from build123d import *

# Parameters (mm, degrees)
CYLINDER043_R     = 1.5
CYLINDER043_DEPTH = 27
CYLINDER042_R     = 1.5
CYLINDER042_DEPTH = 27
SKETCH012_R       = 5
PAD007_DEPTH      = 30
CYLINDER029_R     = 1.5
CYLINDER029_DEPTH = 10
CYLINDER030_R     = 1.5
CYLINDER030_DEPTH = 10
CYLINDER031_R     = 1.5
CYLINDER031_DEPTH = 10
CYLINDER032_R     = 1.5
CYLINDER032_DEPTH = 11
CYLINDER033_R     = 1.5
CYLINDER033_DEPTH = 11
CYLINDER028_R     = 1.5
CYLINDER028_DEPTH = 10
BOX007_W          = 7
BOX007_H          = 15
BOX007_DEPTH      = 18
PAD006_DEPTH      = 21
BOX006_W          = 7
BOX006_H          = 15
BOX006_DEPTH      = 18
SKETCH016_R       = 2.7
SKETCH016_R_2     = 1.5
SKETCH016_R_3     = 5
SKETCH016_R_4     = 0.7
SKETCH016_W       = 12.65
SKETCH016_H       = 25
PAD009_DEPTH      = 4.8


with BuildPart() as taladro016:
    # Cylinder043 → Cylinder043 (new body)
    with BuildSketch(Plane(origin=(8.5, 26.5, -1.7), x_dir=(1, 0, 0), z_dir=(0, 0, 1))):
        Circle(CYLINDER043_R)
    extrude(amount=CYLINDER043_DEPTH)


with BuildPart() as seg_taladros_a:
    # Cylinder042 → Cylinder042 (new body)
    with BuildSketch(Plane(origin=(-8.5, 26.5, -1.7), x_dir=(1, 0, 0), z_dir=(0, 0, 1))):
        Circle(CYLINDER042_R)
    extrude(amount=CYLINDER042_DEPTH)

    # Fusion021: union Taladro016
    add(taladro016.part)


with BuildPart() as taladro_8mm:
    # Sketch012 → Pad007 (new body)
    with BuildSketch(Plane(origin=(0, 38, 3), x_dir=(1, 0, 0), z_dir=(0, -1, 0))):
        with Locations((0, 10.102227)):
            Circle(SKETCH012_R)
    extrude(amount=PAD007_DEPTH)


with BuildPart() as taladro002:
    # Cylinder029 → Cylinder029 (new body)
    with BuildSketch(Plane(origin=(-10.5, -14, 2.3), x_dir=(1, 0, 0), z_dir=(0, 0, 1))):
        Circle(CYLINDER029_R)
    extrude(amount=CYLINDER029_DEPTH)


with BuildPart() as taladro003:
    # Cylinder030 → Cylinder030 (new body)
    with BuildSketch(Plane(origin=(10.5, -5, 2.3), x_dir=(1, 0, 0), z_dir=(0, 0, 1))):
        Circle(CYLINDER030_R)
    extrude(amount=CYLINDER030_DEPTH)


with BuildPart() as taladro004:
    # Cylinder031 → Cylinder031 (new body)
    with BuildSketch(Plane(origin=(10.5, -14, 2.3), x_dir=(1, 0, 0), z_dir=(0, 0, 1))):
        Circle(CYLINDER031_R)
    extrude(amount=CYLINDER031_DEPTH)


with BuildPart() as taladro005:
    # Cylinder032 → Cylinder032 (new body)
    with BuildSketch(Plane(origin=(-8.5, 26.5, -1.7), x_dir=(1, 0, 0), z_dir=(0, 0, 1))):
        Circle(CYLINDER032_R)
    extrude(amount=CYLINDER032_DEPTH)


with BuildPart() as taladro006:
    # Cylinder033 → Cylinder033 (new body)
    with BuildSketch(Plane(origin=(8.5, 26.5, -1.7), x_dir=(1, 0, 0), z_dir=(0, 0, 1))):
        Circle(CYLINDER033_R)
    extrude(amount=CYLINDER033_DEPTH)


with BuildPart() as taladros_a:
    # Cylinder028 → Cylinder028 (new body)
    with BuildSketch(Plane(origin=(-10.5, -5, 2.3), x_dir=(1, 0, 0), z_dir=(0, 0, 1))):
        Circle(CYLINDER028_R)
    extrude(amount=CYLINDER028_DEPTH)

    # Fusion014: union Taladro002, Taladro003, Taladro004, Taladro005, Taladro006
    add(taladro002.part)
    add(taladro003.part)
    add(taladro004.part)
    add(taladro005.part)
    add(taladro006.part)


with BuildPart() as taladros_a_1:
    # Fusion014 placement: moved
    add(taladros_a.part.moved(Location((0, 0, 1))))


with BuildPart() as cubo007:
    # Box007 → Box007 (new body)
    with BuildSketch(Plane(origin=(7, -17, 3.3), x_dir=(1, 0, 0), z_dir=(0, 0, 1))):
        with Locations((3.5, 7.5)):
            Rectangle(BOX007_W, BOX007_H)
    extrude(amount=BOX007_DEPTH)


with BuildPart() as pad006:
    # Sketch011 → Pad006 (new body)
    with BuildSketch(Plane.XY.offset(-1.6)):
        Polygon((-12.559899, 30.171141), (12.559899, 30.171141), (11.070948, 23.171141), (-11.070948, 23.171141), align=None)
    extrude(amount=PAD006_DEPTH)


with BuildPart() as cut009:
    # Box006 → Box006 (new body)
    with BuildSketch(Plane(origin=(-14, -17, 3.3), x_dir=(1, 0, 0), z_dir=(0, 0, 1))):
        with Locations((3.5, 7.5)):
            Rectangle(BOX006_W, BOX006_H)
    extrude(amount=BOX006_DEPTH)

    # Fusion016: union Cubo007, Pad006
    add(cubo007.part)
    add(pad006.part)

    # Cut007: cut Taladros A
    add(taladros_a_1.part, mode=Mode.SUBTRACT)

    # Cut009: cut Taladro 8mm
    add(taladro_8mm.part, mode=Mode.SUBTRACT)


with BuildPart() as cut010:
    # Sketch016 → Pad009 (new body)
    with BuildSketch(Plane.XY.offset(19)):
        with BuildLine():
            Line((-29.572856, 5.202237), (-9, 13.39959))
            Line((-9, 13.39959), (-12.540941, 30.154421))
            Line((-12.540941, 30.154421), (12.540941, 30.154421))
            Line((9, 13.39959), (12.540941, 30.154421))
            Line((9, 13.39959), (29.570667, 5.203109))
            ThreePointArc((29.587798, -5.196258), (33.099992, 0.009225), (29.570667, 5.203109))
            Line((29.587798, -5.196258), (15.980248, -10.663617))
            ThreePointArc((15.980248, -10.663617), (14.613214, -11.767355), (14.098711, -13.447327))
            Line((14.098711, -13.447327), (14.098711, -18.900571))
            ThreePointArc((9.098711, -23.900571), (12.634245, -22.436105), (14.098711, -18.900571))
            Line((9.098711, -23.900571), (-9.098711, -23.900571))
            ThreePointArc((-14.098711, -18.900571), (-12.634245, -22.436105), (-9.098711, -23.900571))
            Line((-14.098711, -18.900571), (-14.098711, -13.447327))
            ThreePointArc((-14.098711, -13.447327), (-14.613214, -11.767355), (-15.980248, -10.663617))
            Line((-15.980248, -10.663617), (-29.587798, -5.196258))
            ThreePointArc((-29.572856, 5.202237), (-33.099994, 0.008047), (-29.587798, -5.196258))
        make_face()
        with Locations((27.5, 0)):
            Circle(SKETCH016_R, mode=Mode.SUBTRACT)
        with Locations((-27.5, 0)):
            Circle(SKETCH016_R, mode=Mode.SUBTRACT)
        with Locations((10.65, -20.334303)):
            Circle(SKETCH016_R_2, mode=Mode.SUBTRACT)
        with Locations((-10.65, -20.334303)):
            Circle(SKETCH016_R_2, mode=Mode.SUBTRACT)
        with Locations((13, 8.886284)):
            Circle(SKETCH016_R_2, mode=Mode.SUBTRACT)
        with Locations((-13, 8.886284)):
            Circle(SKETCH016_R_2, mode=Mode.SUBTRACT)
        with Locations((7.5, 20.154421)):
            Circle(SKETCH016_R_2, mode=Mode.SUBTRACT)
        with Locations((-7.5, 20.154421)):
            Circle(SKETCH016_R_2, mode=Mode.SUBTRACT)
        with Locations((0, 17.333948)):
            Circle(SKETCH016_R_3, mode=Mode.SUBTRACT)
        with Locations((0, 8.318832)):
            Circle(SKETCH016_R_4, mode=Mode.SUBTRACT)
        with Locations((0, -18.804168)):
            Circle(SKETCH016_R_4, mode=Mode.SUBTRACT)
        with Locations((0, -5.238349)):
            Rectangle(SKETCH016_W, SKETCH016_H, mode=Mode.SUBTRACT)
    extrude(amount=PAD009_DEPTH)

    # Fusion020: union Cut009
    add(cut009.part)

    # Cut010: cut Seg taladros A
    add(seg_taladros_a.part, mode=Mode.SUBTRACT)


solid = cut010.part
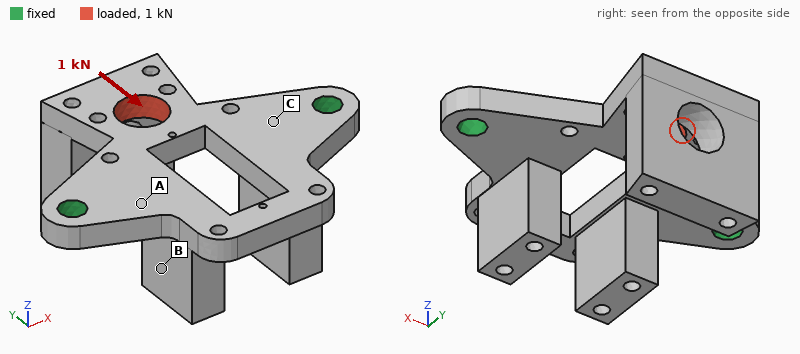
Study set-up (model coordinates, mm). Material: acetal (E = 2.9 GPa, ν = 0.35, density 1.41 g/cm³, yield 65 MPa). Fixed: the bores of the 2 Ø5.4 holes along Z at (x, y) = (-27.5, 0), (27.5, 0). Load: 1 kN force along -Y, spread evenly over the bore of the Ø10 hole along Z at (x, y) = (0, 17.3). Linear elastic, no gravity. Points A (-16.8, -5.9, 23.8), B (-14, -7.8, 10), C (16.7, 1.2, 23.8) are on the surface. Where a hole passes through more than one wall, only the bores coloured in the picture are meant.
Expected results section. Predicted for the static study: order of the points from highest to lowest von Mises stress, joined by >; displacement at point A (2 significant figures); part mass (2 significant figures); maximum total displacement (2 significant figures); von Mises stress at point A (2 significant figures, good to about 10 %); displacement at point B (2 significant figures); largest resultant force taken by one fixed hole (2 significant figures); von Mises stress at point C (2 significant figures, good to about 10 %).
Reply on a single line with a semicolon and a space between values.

C > A > B; 0.14 mm; 18 g; 0.32 mm; 8.7 MPa; 0.19 mm; 580 N; 12 MPa
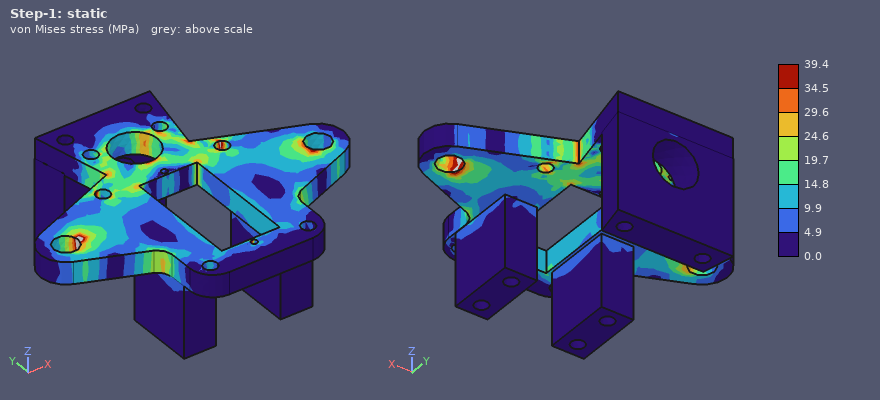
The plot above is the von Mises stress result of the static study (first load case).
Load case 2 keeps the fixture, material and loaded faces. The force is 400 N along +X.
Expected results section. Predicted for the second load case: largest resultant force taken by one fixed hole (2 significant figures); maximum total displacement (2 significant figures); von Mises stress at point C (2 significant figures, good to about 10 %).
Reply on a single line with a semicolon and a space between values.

240 N; 0.25 mm; 3.5 MPa
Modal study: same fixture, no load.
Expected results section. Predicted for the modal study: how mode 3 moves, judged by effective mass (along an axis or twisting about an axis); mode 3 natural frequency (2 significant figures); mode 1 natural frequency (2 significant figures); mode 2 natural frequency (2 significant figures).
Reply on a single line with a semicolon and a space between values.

along Z; 990 Hz; 380 Hz; 760 Hz
